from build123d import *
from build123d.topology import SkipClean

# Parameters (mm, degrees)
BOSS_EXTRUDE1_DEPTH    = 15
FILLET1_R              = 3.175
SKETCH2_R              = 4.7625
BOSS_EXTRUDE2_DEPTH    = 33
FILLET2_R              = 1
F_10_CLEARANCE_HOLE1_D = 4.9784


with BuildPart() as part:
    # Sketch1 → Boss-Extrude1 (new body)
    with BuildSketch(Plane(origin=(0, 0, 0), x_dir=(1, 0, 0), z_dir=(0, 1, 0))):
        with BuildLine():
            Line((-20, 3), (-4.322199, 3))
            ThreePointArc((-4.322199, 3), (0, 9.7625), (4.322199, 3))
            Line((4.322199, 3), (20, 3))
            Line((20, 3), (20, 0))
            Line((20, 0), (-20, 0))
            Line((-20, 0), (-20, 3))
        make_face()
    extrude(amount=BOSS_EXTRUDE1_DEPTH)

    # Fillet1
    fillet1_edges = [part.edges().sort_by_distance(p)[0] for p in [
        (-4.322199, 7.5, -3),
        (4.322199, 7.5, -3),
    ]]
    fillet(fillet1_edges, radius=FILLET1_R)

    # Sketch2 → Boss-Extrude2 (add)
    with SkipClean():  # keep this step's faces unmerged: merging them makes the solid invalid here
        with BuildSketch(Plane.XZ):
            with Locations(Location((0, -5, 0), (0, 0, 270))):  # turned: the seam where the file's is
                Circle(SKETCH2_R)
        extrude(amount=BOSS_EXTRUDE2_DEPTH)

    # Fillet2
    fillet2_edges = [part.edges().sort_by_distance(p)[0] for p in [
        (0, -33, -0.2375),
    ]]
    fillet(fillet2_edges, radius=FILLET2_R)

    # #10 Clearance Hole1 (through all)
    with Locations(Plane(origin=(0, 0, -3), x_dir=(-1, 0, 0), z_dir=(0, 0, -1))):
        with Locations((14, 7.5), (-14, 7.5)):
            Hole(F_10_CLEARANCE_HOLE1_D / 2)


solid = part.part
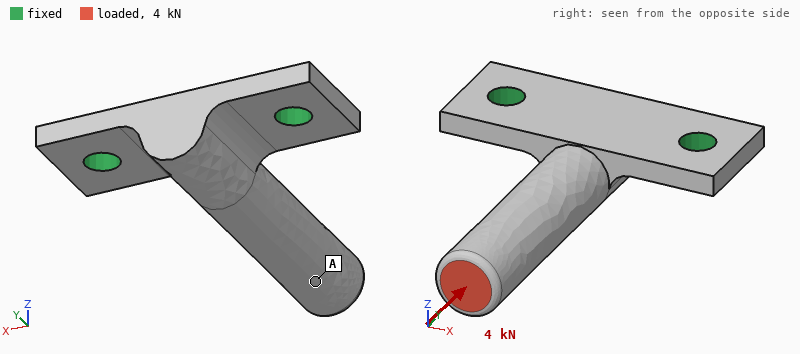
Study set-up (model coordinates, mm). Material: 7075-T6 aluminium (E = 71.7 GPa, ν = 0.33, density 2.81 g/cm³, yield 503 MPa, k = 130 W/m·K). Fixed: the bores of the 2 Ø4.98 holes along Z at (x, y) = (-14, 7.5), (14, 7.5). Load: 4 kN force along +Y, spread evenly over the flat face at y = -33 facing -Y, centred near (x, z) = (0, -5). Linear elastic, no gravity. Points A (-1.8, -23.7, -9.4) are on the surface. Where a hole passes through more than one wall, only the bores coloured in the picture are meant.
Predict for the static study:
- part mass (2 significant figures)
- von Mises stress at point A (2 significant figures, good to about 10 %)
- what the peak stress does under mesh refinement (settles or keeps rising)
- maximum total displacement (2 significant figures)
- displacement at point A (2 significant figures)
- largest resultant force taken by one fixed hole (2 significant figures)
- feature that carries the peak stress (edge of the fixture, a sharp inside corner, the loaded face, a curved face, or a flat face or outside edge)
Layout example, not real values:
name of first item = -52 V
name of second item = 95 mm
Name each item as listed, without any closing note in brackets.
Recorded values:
part mass = 14 g
von Mises stress at point A = 56 MPa
what the peak stress does under mesh refinement = keeps rising
maximum total displacement = 0.48 mm
displacement at point A = 0.38 mm
largest resultant force taken by one fixed hole = 2.0 kN
feature that carries the peak stress = edge of the fixture
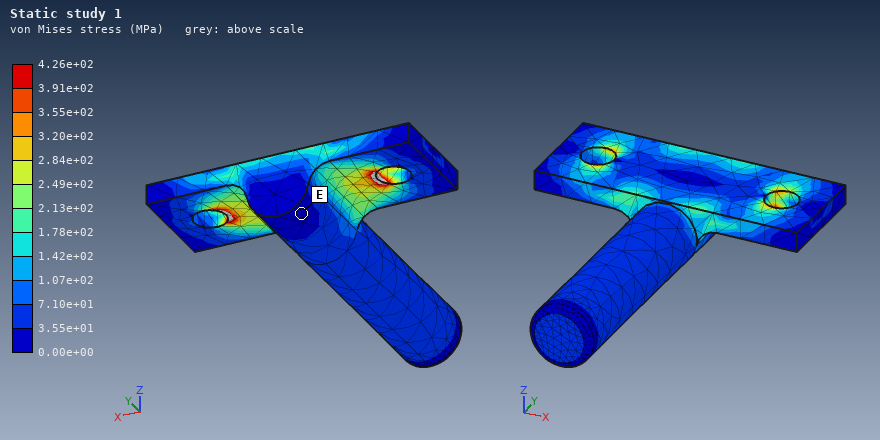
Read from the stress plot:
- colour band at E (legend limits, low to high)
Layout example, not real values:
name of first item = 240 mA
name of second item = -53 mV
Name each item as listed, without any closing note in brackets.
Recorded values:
colour band at E = 0.00e+00 to 3.55e+01 MPa
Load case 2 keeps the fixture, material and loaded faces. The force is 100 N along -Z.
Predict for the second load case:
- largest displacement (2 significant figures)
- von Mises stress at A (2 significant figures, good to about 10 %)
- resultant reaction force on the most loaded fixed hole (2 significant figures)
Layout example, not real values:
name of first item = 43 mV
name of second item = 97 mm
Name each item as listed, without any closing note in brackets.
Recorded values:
largest displacement = 0.19 mm
von Mises stress at A = 10 MPa
resultant reaction force on the most loaded fixed hole = 95 N
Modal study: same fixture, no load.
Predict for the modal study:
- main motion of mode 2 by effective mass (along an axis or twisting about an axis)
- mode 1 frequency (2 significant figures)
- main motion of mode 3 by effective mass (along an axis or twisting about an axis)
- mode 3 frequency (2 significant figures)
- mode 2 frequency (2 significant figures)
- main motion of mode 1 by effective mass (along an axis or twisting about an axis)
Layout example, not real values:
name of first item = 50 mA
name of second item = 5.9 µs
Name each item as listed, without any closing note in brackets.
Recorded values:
main motion of mode 2 by effective mass = along X
mode 1 frequency = 2400 Hz
main motion of mode 3 by effective mass = along Y
mode 3 frequency = 14 kHz
mode 2 frequency = 4600 Hz
main motion of mode 1 by effective mass = along Z
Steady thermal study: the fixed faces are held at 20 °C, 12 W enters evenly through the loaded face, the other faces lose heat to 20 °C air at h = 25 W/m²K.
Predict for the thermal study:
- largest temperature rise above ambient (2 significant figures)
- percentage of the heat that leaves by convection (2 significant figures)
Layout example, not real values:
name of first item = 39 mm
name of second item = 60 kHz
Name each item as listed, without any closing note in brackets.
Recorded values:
largest temperature rise above ambient = 56 K
percentage of the heat that leaves by convection = 8.6 %
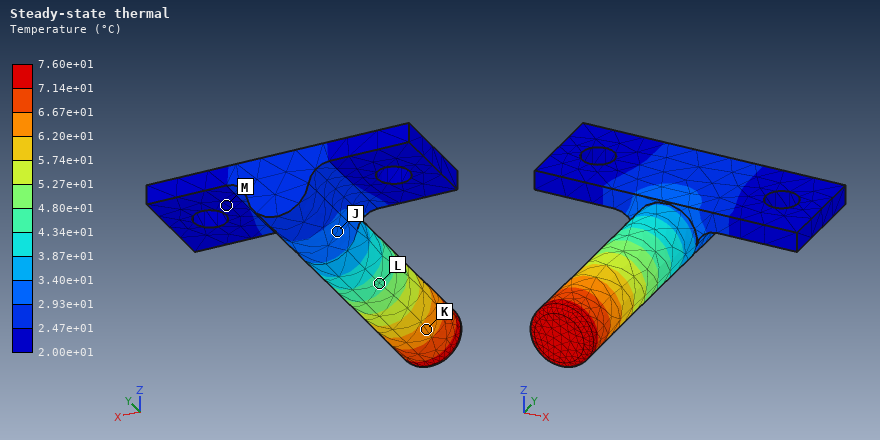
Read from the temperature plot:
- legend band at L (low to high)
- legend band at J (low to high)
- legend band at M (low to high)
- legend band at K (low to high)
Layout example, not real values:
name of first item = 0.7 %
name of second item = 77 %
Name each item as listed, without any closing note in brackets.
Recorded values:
legend band at L = 4.34e+01 to 4.80e+01 °C
legend band at J = 2.93e+01 to 3.40e+01 °C
legend band at M = 2.00e+01 to 2.47e+01 °C
legend band at K = 6.20e+01 to 6.67e+01 °C
